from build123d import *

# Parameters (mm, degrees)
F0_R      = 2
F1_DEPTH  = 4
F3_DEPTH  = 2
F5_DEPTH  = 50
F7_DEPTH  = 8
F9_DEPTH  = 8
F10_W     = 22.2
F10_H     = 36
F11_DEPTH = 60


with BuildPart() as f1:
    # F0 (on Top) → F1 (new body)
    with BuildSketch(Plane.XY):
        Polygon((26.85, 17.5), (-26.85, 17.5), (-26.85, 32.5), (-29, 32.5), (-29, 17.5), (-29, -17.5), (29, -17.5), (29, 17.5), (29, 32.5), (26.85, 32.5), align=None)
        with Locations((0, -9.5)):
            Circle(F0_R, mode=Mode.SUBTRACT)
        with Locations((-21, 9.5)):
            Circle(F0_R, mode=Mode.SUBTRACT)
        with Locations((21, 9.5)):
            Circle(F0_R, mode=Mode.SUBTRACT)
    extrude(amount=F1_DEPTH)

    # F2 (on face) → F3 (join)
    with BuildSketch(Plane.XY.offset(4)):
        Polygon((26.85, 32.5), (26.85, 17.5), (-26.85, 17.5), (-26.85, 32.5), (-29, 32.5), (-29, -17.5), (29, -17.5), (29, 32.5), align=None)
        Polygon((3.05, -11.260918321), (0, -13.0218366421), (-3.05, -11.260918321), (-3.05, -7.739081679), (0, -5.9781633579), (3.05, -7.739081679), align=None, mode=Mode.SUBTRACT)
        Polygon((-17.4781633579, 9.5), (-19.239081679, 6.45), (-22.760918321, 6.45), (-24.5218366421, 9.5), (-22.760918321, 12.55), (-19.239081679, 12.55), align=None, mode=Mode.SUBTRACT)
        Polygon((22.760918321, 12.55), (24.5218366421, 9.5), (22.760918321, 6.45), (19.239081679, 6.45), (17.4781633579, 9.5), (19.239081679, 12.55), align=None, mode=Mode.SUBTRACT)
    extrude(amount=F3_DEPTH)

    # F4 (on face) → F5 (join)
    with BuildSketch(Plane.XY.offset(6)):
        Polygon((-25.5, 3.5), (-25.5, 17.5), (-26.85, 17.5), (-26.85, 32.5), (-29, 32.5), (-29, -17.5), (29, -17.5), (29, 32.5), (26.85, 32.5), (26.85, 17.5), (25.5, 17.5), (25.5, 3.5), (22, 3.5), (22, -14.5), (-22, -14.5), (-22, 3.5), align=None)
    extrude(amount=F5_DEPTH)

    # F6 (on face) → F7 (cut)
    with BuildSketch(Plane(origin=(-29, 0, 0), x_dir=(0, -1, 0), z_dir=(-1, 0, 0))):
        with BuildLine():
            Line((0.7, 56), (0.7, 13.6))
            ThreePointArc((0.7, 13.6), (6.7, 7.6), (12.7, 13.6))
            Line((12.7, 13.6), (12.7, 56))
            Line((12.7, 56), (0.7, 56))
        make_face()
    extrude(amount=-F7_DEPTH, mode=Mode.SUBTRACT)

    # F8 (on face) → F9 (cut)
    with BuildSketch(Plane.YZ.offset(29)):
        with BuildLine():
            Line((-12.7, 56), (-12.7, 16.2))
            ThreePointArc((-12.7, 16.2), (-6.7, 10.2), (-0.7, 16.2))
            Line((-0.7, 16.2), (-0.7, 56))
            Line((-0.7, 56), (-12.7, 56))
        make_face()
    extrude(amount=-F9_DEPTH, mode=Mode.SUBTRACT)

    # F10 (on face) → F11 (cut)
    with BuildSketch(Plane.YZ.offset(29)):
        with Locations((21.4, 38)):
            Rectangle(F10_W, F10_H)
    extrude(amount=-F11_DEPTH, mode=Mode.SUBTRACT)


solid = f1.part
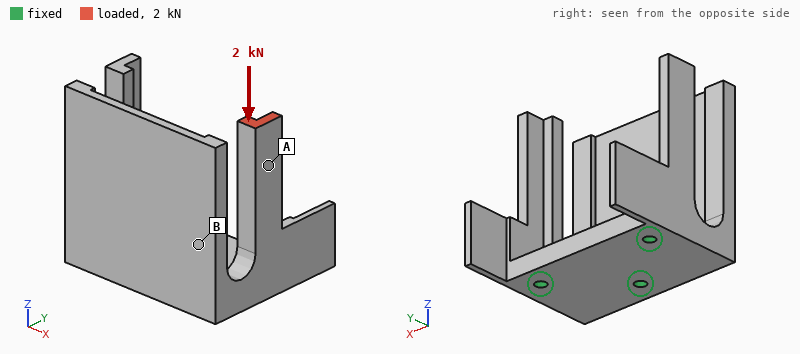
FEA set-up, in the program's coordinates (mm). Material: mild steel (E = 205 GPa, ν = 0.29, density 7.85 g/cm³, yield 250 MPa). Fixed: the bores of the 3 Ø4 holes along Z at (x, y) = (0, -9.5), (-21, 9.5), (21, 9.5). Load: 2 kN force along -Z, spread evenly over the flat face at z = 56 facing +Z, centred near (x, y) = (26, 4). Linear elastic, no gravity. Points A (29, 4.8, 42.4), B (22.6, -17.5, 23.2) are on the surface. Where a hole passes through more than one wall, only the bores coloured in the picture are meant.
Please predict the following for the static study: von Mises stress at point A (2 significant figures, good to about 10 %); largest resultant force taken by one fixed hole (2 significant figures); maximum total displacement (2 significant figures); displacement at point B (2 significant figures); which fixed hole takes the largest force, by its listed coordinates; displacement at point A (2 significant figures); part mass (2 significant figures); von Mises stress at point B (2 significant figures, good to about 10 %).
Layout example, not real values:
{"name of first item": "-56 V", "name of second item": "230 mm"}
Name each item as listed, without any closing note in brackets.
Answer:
{"von Mises stress at point A": "38 MPa", "largest resultant force taken by one fixed hole": "1.8 kN", "maximum total displacement": "47 µm", "displacement at point B": "12 µm", "which fixed hole takes the largest force, by its listed coordinates": "(21, 9.5)", "displacement at point A": "35 µm", "part mass": "230 g", "von Mises stress at point B": "7.1 MPa"}
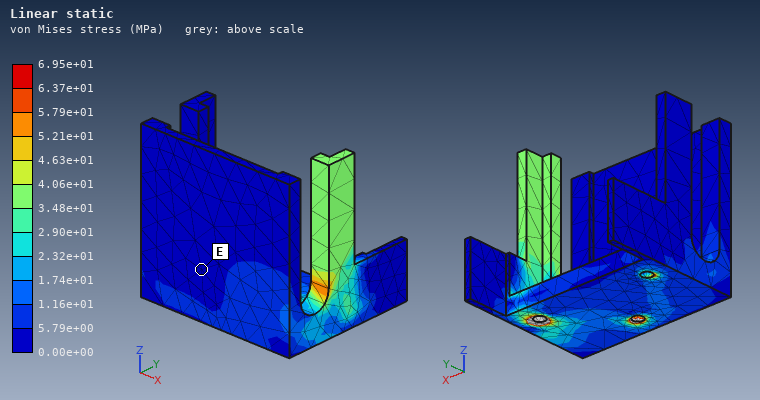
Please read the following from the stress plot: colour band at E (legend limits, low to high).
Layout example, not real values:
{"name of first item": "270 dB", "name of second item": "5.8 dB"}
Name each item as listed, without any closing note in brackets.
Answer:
{"colour band at E": "0.00e+00 to 5.79e+00 MPa"}
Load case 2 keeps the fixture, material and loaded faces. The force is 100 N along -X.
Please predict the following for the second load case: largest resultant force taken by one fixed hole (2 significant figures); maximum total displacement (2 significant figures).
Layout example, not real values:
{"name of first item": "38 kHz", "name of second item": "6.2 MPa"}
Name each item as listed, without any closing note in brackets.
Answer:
{"largest resultant force taken by one fixed hole": "94 N", "maximum total displacement": "0.14 mm"}
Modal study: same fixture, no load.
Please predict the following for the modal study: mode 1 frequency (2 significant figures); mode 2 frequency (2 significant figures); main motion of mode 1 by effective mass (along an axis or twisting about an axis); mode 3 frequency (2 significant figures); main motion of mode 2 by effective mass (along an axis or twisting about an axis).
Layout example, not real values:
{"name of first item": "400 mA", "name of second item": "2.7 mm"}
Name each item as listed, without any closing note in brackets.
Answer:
{"mode 1 frequency": "1300 Hz", "mode 2 frequency": "1700 Hz", "main motion of mode 1 by effective mass": "along Y", "mode 3 frequency": "1900 Hz", "main motion of mode 2 by effective mass": "along X"}
